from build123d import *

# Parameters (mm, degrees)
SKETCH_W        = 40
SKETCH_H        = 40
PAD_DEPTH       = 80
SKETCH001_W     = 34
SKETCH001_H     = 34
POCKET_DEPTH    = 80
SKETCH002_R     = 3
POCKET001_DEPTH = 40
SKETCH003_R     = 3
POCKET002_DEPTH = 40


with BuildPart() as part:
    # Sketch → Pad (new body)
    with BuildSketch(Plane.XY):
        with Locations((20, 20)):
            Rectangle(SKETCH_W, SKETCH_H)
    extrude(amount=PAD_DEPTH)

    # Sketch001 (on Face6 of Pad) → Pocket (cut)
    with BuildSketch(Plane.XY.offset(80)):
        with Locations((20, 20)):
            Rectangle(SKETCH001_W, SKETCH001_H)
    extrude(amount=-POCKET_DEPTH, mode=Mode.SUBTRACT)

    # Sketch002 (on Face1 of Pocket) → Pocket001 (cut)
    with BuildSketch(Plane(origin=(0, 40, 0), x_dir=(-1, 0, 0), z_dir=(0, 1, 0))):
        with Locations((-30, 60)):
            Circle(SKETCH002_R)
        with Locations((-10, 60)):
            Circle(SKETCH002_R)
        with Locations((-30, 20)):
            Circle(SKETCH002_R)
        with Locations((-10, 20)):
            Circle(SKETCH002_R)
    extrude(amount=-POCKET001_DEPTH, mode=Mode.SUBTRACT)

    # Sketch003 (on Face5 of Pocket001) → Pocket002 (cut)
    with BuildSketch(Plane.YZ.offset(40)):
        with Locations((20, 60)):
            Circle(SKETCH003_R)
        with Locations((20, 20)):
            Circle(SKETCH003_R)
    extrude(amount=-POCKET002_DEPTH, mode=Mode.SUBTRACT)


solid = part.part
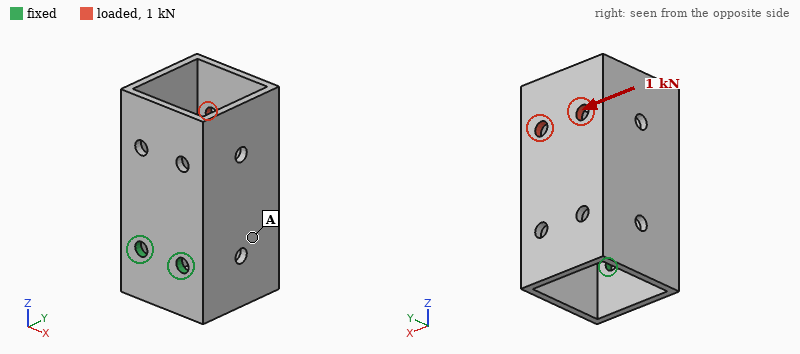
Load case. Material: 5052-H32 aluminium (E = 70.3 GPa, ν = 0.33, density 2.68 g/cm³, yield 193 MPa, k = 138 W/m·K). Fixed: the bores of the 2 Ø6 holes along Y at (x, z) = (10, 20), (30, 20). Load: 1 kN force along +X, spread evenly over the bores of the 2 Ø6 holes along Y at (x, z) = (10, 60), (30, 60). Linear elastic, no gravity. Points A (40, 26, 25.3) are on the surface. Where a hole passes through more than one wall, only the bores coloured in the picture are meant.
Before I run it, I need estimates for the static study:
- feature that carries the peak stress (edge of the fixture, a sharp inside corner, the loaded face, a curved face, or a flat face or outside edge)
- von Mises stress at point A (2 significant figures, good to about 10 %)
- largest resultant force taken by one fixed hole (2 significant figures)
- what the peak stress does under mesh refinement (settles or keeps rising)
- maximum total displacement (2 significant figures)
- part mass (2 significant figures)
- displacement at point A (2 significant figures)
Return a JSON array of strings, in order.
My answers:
["edge of the fixture", "22 MPa", "2.0 kN", "keeps rising", "0.46 mm", "92 g", "0.31 mm"]
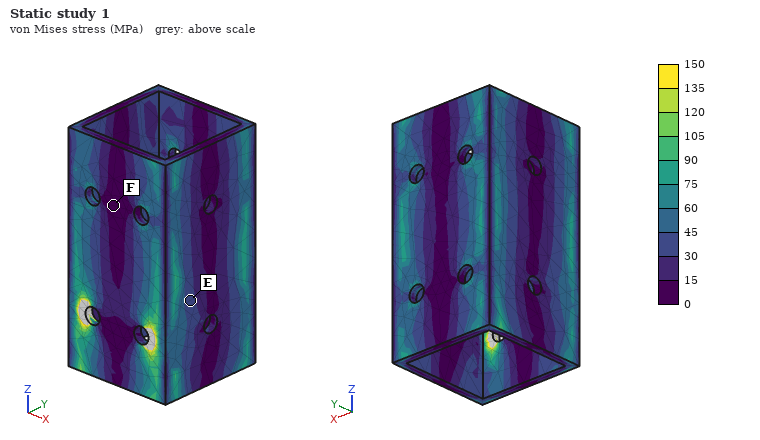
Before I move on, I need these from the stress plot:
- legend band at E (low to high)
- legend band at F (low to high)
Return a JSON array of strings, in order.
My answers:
["30 to 45 MPa", "0 to 15 MPa"]
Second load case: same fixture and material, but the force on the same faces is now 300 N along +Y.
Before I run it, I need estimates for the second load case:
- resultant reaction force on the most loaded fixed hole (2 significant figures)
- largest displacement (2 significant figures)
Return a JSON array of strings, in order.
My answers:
["150 N", "0.28 mm"]
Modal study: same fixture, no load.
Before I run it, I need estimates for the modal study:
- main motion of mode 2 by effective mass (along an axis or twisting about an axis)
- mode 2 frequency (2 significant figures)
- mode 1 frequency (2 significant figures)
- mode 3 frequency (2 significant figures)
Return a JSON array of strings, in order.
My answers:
["along X", "1100 Hz", "770 Hz", "2400 Hz"]
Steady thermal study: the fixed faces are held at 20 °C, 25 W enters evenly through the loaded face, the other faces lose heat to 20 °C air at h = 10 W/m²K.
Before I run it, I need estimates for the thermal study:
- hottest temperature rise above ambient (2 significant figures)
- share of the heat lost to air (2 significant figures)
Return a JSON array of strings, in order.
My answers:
["42 K", "18 %"]
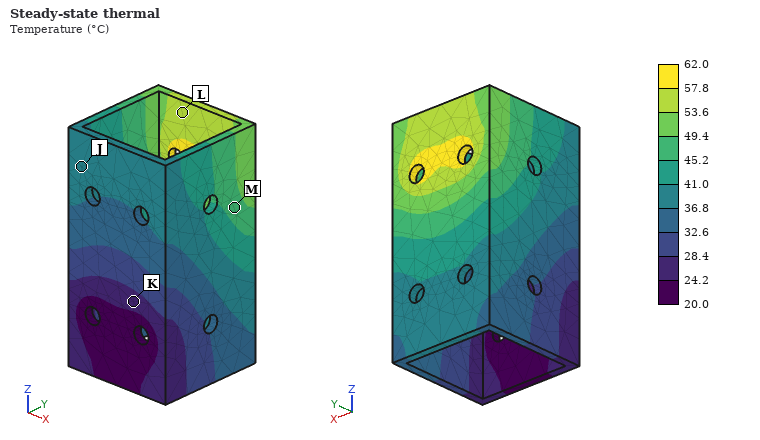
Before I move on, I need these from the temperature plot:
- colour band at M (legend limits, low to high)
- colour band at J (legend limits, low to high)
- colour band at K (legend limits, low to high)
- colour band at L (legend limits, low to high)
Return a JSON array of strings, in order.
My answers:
["45.2 to 49.4 °C", "36.8 to 41.0 °C", "24.2 to 28.4 °C", "53.6 to 57.8 °C"]
